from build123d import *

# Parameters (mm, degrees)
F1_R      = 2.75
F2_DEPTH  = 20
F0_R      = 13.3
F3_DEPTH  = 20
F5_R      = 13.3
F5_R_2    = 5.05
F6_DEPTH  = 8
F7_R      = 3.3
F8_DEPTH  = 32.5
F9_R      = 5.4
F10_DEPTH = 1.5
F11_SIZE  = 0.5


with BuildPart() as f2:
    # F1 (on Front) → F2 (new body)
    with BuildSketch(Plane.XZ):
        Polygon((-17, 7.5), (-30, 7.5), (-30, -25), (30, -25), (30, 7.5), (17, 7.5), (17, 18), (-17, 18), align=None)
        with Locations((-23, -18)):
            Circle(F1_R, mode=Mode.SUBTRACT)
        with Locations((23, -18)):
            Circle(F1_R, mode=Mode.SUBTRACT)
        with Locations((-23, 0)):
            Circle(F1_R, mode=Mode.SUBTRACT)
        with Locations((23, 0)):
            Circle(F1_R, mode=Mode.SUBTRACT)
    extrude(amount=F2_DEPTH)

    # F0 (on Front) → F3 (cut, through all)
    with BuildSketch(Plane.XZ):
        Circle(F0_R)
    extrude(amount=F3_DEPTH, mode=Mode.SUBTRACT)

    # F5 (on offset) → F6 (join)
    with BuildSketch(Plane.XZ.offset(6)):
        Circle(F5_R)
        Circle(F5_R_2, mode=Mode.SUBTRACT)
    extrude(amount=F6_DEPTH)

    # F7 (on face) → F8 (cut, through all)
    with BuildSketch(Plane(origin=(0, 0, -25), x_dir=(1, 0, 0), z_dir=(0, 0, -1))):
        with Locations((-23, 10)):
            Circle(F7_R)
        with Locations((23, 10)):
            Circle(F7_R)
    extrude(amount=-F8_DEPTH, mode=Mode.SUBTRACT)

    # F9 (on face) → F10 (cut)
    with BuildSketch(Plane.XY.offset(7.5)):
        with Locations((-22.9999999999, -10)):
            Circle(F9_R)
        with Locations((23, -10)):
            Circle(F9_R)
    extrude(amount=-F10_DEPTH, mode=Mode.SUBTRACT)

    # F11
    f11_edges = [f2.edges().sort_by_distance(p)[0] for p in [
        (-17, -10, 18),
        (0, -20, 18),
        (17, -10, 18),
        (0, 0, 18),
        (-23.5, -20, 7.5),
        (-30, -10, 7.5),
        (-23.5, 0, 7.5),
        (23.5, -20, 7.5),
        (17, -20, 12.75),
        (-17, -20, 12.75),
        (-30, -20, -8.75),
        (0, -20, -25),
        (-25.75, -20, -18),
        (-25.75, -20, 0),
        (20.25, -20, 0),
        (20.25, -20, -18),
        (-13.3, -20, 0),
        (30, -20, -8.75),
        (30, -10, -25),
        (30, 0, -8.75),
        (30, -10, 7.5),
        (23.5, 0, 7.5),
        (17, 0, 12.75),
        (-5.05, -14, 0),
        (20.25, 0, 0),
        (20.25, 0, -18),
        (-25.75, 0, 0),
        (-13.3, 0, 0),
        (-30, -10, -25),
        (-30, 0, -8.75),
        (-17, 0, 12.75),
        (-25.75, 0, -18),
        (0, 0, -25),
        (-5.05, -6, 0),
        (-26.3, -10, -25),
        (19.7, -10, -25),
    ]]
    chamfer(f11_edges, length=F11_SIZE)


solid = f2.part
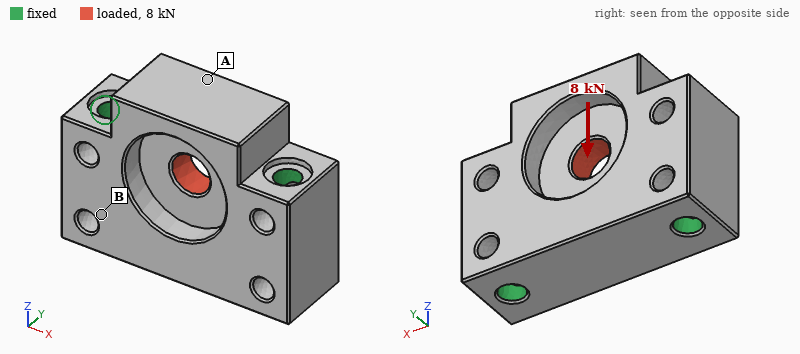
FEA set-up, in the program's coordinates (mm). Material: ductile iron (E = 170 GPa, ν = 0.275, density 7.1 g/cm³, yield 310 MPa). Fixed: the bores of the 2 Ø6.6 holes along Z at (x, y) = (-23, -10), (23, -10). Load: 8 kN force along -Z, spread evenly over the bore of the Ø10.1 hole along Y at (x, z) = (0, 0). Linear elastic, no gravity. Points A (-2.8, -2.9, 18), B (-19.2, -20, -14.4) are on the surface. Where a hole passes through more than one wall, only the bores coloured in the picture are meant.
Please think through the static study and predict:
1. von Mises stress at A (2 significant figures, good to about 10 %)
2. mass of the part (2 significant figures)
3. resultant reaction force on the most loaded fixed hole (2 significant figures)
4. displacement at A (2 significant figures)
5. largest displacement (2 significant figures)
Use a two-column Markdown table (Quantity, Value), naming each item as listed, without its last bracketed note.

| Quantity | Value |
|---|---|
| von Mises stress at A | 16 MPa |
| mass of the part | 250 g |
| resultant reaction force on the most loaded fixed hole | 4.1 kN |
| displacement at A | 2.5 µm |
| largest displacement | 4.2 µm |
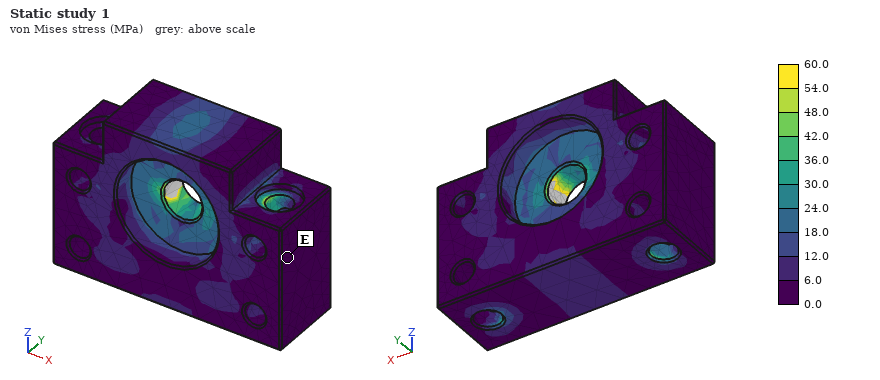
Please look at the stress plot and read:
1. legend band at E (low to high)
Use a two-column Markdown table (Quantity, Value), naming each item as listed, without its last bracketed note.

| Quantity | Value |
|---|---|
| legend band at E | 0.0 to 6.0 MPa |
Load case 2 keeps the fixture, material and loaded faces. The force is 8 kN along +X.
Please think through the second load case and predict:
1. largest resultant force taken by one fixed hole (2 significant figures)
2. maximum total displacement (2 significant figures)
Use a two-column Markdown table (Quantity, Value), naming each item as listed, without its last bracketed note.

| Quantity | Value |
|---|---|
| largest resultant force taken by one fixed hole | 4.1 kN |
| maximum total displacement | 3.2 µm |
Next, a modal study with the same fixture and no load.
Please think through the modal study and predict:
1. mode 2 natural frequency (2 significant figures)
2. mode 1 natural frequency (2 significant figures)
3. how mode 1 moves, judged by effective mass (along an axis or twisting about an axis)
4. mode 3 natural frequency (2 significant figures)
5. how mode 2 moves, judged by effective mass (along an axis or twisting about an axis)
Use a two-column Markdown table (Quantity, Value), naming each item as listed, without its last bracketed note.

| Quantity | Value |
|---|---|
| mode 2 natural frequency | 24 kHz |
| mode 1 natural frequency | 15 kHz |
| how mode 1 moves, judged by effective mass | along Y |
| mode 3 natural frequency | 26 kHz |
| how mode 2 moves, judged by effective mass | along Y |
